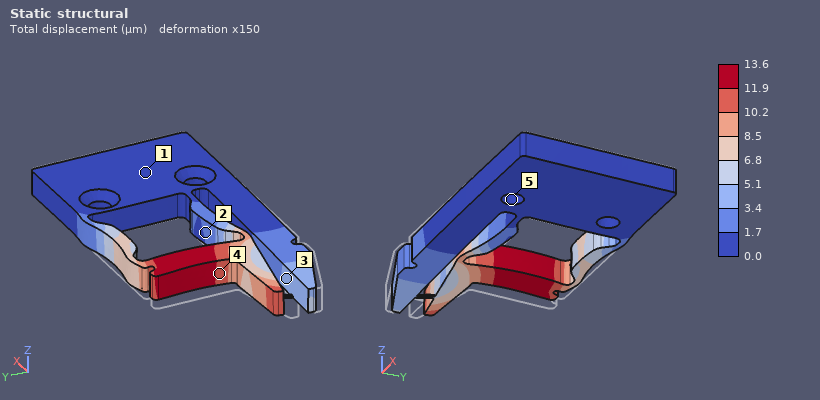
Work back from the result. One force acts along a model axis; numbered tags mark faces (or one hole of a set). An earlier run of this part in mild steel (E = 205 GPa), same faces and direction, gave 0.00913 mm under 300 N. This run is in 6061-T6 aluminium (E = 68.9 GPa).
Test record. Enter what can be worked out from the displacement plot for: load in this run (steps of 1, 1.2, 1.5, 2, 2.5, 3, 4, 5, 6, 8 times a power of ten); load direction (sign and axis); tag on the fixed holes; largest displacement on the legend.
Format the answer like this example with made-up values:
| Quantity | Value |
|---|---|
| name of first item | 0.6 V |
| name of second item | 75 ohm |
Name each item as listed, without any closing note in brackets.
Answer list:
| Quantity | Value |
|---|---|
| load in this run | 150 N |
| load direction | +X |
| tag on the fixed holes | 5 |
| largest displacement on the legend | 13.6 µm |
